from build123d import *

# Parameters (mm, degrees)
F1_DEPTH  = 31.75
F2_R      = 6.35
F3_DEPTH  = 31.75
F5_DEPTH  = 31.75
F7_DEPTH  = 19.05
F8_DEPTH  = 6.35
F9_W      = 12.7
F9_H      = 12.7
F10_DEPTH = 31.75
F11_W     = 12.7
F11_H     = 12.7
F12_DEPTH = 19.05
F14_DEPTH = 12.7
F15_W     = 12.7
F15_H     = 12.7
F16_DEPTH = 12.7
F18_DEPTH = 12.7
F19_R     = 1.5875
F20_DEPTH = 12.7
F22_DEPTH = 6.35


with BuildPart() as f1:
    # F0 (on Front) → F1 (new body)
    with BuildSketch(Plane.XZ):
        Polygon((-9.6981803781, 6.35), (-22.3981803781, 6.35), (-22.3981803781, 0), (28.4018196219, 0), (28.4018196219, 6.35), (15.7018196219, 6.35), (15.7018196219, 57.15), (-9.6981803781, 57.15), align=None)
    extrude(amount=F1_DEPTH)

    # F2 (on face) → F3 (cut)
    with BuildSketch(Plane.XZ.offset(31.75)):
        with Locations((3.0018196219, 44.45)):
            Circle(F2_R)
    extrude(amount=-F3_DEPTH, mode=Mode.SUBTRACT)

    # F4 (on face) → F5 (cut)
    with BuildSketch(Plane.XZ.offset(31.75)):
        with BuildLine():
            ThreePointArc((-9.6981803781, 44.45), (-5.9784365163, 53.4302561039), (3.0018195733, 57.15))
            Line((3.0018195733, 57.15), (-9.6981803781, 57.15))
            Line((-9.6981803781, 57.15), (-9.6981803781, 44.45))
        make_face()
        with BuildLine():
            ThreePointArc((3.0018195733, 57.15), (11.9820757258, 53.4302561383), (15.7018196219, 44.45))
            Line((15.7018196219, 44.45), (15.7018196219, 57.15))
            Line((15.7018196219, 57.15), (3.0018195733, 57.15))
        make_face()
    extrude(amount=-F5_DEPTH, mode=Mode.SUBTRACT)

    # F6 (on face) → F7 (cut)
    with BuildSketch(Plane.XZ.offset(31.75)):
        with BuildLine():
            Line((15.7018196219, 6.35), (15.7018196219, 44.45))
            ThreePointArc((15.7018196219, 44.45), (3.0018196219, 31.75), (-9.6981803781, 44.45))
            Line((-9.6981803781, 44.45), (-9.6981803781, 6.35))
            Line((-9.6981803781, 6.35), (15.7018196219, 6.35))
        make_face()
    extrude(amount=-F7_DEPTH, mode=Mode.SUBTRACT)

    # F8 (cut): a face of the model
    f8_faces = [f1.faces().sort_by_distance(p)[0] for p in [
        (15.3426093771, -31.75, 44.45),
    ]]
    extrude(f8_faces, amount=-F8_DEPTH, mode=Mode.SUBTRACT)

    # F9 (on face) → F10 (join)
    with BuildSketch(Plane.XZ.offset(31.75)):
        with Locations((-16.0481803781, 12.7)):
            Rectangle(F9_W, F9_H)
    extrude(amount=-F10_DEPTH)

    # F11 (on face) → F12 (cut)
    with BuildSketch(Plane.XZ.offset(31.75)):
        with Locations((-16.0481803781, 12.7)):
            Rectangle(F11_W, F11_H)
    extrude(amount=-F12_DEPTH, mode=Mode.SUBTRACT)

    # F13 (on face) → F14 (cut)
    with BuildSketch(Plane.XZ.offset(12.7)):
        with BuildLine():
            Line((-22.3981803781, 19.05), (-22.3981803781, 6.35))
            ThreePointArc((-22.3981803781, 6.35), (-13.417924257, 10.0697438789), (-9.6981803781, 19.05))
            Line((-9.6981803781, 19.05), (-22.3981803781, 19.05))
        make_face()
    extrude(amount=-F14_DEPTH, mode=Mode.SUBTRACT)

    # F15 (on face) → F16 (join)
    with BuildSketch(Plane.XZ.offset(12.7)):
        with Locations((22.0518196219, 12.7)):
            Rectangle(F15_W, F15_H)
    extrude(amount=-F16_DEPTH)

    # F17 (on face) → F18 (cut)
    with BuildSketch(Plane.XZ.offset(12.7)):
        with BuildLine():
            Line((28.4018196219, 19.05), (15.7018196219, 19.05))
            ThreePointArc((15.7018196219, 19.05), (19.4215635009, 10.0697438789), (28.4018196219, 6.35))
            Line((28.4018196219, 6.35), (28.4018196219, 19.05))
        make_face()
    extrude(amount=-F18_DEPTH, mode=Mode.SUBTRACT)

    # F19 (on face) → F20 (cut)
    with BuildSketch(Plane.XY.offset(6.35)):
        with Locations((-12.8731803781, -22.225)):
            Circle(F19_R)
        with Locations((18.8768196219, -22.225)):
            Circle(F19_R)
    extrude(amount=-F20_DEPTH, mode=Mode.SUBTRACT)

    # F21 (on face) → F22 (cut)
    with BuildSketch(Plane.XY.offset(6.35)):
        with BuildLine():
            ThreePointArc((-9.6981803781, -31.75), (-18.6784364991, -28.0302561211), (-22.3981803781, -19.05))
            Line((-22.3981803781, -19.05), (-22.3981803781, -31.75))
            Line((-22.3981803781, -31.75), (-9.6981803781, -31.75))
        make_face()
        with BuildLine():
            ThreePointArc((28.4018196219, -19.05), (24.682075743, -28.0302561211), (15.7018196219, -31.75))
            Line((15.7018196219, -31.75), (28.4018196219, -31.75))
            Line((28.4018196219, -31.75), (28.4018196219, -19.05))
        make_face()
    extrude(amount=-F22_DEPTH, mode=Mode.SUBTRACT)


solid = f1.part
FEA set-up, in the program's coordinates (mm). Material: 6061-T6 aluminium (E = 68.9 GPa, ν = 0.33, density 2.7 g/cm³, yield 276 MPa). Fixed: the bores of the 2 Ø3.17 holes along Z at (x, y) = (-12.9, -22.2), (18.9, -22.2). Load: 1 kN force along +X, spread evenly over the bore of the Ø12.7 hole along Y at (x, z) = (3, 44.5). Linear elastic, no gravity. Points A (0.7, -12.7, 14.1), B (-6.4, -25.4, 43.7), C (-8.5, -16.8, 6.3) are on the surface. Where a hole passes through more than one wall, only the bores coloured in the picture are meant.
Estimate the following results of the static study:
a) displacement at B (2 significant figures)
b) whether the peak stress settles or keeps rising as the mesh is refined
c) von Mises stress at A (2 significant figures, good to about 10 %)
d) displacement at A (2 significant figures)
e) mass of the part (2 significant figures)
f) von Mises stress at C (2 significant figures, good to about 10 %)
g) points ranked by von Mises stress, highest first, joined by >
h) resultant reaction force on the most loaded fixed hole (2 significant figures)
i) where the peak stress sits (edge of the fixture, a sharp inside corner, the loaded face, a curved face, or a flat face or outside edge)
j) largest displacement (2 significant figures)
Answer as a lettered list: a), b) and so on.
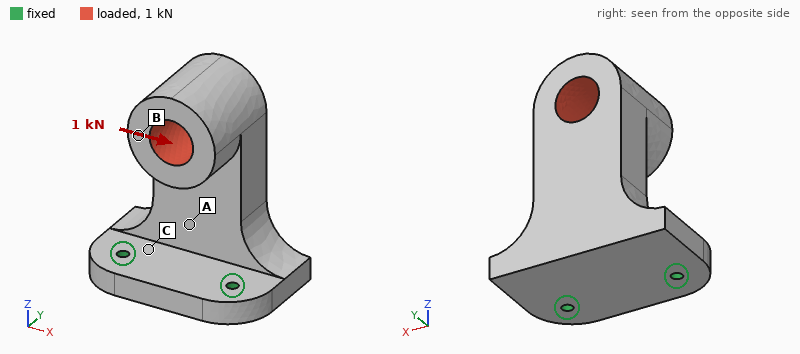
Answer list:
a) 0.094 mm
b) keeps rising
c) 20 MPa
d) 0.019 mm
e) 79 g
f) 33 MPa
g) C > A > B
h) 1.3 kN
i) edge of the fixture
j) 0.12 mm
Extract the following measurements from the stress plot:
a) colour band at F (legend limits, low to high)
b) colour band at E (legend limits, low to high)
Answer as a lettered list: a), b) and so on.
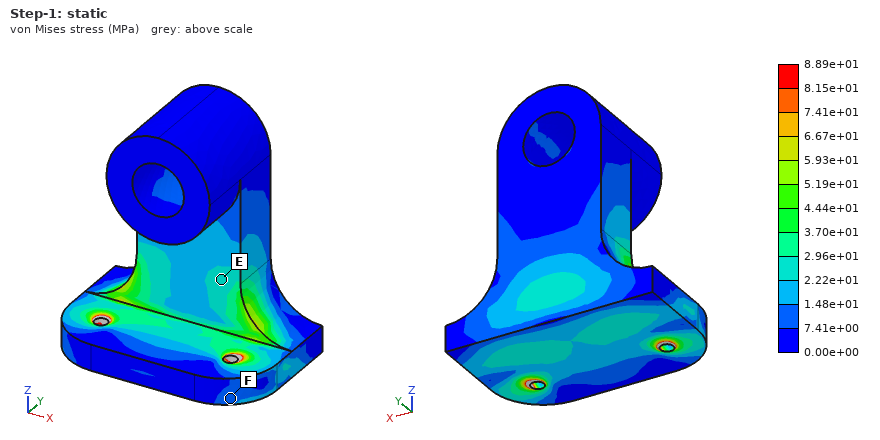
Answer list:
a) 7.41e+00 to 1.48e+01 MPa
b) 2.22e+01 to 2.96e+01 MPa
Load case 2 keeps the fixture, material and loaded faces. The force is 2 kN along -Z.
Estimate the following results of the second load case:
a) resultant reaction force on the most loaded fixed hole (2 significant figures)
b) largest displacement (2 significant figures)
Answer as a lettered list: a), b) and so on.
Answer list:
a) 1.0 kN
b) 67 µm
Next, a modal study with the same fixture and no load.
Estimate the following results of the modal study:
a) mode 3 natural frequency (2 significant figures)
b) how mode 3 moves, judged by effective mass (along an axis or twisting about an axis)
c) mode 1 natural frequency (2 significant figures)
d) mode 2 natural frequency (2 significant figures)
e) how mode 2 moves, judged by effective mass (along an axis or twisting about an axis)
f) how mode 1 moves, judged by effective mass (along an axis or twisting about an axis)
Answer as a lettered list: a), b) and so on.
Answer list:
a) 5700 Hz
b) along Z
c) 1300 Hz
d) 3100 Hz
e) along X
f) along Y
